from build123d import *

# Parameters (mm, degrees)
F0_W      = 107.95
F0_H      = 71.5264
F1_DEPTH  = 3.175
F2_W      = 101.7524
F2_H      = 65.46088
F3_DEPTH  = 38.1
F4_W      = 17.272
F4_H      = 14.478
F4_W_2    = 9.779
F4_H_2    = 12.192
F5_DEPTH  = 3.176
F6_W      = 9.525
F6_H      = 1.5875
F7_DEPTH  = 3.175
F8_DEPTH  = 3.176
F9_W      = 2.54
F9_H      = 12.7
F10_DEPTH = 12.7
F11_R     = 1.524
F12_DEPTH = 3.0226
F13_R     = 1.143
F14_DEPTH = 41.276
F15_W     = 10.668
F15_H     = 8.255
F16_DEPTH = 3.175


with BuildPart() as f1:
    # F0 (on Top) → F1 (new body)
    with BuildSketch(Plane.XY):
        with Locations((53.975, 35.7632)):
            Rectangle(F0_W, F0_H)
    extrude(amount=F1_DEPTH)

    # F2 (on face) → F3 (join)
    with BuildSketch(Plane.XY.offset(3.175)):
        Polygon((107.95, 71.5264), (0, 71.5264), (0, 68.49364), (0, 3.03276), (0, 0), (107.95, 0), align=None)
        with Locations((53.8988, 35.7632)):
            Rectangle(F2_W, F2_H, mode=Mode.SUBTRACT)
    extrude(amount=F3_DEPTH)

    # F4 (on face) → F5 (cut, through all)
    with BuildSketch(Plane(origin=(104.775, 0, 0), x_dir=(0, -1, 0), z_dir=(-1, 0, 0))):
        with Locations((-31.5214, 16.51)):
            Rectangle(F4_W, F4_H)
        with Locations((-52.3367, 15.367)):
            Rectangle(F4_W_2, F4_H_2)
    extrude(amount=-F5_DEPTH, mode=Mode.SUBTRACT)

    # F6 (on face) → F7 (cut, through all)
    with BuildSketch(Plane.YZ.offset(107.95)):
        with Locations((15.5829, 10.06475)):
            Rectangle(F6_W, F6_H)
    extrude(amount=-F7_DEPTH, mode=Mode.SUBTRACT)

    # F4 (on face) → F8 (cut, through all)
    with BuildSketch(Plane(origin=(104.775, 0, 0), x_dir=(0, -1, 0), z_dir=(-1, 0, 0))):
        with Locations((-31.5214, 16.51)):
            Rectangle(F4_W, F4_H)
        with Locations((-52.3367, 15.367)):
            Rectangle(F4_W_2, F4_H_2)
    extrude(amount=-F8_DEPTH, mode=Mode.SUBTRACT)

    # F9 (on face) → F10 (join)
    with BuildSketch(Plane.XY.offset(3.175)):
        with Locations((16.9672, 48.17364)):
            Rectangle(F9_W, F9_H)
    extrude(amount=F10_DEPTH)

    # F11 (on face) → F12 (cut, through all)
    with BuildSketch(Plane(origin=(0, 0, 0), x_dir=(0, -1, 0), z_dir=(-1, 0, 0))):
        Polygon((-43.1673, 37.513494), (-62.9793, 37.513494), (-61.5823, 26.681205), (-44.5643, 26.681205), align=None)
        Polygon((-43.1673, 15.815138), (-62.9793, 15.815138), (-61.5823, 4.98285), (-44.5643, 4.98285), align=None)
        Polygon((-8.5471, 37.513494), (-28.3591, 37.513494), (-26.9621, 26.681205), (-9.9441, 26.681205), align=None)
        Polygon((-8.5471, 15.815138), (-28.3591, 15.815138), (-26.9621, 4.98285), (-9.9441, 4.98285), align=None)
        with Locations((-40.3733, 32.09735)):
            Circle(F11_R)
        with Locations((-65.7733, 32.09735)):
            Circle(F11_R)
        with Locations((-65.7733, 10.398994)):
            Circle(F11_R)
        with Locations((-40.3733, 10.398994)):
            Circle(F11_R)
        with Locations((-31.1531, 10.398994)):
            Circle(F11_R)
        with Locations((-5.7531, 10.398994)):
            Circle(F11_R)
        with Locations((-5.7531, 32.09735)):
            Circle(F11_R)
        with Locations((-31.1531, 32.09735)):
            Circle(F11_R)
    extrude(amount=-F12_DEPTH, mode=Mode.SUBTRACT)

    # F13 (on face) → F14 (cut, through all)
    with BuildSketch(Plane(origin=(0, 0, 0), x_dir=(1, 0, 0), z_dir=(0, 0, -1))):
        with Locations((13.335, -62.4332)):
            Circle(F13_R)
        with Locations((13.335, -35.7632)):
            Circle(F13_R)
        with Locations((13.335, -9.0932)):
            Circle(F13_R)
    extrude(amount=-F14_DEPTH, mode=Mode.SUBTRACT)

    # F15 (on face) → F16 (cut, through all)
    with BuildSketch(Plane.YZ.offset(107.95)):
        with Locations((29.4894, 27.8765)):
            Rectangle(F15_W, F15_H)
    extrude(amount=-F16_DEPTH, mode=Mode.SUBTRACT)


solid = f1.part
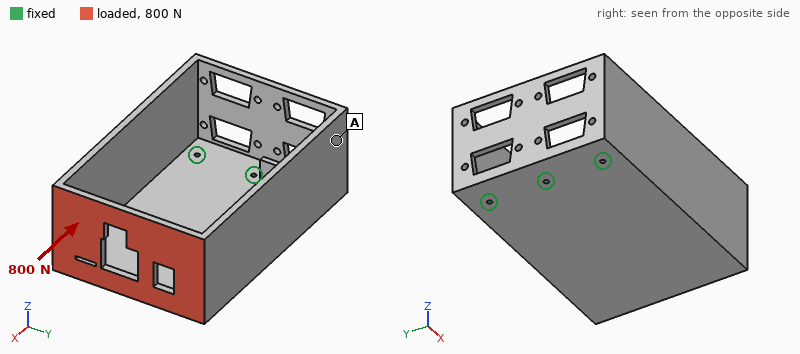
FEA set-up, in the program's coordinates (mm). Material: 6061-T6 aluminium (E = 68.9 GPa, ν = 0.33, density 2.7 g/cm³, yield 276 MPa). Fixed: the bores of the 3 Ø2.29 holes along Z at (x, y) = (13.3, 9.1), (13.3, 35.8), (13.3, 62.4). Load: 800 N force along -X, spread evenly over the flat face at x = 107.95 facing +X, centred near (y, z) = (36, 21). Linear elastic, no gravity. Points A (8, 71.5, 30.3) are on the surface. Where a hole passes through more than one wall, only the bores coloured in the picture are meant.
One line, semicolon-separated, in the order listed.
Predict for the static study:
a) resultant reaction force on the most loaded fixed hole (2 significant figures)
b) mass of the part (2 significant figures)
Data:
370 N; 170 g
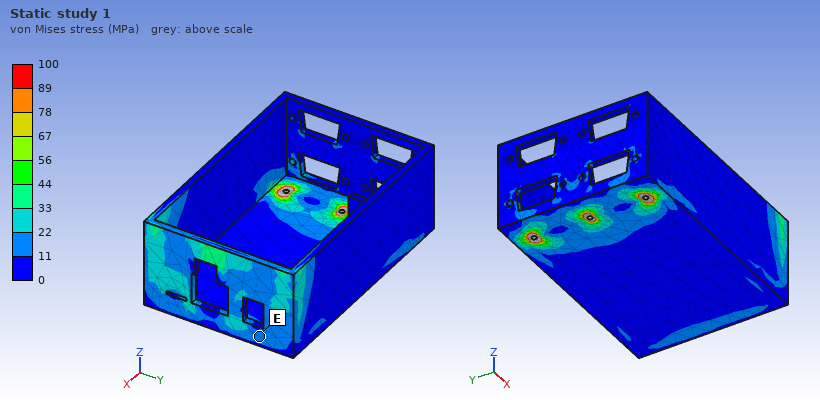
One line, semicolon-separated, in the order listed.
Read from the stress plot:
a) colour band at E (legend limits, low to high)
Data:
11 to 22 MPa
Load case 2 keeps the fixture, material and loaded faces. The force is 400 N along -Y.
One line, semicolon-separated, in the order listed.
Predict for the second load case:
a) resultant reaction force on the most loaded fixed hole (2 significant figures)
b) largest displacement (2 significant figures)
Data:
730 N; 0.45 mm
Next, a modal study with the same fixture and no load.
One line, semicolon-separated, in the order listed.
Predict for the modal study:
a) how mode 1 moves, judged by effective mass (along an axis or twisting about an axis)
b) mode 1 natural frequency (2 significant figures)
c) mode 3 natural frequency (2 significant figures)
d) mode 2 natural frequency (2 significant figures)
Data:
along Z; 330 Hz; 1900 Hz; 600 Hz
